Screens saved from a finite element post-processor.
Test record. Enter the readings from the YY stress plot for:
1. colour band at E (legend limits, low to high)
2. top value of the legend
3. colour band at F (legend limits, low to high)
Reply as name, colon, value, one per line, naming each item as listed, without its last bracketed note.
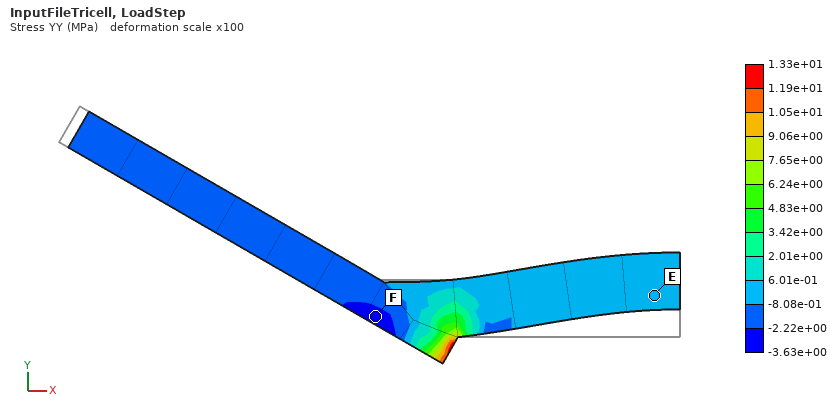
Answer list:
colour band at E: -8.08e-01 to 6.01e-01 MPa
top value of the legend: 1.33e+01 MPa
colour band at F: -3.63e+00 to -2.22e+00 MPa
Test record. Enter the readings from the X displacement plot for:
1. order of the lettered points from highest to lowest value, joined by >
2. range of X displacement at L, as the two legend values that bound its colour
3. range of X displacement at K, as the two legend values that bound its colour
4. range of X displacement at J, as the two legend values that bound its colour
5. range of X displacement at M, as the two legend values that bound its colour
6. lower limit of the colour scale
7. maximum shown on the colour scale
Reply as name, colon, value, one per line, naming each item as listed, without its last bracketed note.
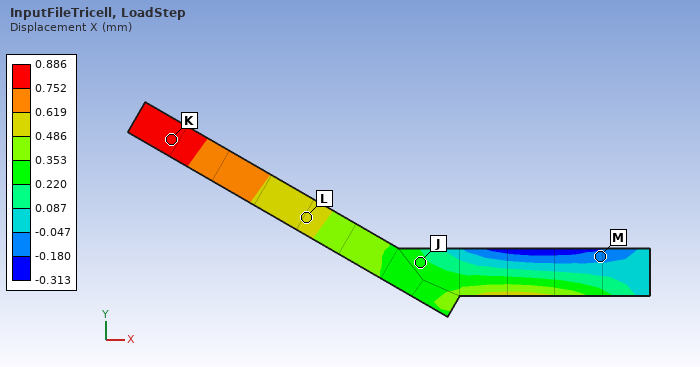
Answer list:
order of the lettered points from highest to lowest value, joined by >: K > L > J > M
range of X displacement at L, as the two legend values that bound its colour: 0.486 to 0.619 mm
range of X displacement at K, as the two legend values that bound its colour: 0.752 to 0.886 mm
range of X displacement at J, as the two legend values that bound its colour: 0.220 to 0.353 mm
range of X displacement at M, as the two legend values that bound its colour: -0.180 to -0.047 mm
lower limit of the colour scale: -0.313 mm
maximum shown on the colour scale: 0.886 mm
